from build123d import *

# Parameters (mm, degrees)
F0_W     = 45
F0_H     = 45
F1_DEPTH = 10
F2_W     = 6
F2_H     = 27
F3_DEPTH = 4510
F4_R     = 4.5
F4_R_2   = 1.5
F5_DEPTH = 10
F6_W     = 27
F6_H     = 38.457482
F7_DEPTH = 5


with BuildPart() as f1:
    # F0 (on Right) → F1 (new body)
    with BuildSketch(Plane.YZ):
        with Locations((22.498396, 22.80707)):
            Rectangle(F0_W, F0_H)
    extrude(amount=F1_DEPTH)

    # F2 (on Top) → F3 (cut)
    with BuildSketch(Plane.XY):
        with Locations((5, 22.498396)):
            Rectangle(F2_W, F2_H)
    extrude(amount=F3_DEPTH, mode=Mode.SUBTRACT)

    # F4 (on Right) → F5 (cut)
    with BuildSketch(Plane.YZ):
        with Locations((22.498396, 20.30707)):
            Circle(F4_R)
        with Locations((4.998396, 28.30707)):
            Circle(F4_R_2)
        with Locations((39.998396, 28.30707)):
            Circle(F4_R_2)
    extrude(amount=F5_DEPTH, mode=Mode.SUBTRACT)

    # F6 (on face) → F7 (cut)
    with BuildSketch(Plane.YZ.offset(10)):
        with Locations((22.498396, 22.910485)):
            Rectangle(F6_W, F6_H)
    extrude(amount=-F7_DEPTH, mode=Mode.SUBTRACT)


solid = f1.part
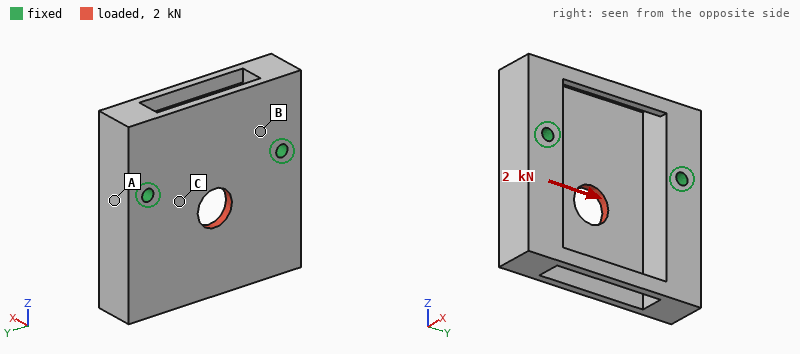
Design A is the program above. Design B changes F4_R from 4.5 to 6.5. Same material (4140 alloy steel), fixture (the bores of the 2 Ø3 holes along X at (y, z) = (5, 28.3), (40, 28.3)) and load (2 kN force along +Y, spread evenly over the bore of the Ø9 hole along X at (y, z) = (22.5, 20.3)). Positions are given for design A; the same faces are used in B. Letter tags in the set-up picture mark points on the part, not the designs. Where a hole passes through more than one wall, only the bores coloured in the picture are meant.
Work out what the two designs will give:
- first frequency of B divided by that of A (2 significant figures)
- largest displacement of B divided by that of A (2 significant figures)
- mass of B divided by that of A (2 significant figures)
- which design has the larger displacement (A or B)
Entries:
1.0
1.1
0.99
B
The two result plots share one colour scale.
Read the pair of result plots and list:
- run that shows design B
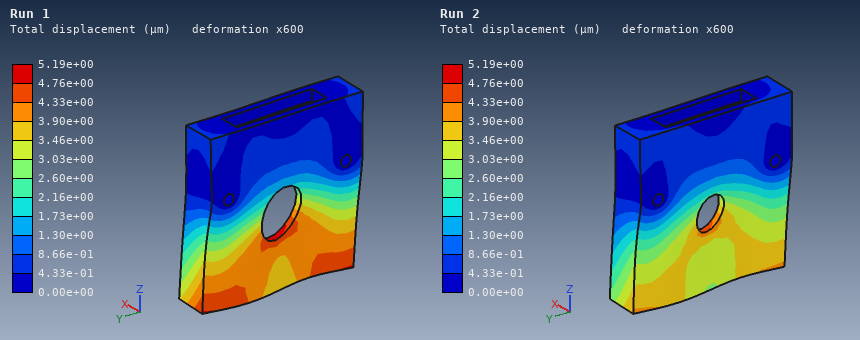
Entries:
Run 1
